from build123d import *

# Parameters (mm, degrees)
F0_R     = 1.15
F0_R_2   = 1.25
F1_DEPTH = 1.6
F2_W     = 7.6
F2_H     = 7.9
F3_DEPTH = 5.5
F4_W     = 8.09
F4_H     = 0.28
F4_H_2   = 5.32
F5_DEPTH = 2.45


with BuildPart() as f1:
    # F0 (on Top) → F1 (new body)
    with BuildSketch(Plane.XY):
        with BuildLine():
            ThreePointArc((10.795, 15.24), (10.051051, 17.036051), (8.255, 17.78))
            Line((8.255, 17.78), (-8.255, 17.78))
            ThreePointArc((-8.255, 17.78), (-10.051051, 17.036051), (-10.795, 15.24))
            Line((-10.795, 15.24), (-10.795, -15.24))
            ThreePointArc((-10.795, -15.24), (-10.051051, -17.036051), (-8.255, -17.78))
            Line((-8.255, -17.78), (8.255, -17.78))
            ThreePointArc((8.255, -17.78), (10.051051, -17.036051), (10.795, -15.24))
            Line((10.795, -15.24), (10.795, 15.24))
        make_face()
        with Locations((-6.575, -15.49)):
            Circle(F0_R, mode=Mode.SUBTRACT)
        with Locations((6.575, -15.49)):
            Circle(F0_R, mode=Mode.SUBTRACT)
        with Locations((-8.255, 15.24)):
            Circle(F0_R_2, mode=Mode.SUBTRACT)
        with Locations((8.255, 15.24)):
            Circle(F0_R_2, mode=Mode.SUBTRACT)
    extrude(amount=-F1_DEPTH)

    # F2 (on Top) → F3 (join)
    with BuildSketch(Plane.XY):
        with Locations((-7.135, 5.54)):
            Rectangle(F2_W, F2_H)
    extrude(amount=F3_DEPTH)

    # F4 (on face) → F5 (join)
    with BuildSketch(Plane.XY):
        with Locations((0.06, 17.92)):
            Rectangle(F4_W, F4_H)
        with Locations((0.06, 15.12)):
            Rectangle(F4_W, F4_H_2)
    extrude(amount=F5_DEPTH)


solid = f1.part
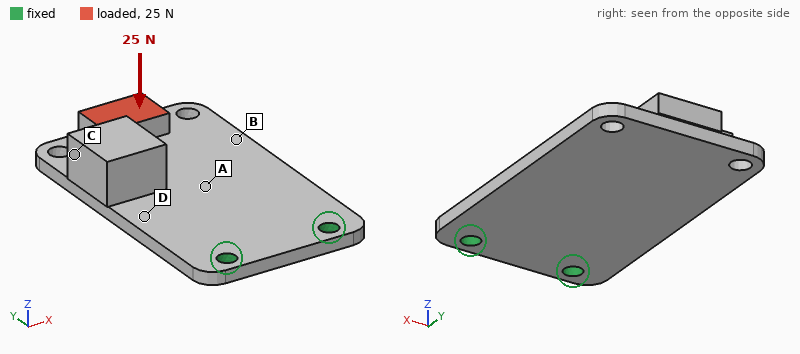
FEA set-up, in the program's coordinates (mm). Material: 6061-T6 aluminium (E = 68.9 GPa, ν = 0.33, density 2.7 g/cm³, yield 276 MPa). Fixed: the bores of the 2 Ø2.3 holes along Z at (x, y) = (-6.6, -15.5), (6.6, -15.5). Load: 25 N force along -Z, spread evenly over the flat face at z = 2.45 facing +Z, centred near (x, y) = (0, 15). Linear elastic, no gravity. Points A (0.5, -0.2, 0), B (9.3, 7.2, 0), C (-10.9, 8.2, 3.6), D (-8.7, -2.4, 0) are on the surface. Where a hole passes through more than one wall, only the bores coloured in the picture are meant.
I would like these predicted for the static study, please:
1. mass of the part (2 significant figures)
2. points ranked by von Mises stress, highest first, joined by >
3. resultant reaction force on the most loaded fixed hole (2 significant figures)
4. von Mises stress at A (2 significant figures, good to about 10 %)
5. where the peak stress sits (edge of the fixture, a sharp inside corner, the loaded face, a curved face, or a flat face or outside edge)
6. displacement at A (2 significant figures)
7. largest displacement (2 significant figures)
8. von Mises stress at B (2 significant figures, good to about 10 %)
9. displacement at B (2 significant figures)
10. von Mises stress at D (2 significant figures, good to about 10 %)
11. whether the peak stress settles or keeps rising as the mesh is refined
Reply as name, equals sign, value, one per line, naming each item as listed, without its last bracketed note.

mass of the part = 4.4 g
points ranked by von Mises stress, highest first, joined by > = D > A > B > C
resultant reaction force on the most loaded fixed hole = 13 N
von Mises stress at A = 38 MPa
where the peak stress sits = edge of the fixture
displacement at A = 0.15 mm
largest displacement = 0.51 mm
von Mises stress at B = 17 MPa
displacement at B = 0.28 mm
von Mises stress at D = 50 MPa
whether the peak stress settles or keeps rising as the mesh is refined = keeps rising
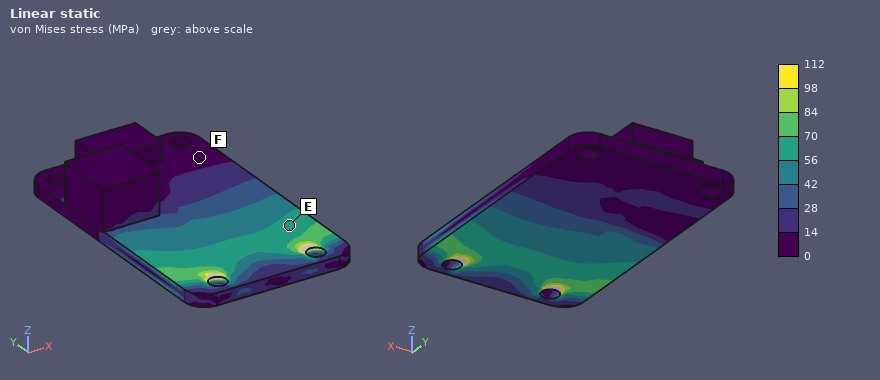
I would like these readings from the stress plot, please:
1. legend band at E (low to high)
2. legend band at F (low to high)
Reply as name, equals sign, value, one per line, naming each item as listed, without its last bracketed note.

legend band at E = 56 to 70 MPa
legend band at F = 0 to 14 MPa
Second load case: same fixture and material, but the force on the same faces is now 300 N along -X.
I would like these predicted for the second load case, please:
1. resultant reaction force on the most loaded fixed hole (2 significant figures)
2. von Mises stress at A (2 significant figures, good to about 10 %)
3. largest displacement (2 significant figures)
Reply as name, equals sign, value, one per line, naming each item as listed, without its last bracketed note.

resultant reaction force on the most loaded fixed hole = 650 N
von Mises stress at A = 92 MPa
largest displacement = 0.26 mm
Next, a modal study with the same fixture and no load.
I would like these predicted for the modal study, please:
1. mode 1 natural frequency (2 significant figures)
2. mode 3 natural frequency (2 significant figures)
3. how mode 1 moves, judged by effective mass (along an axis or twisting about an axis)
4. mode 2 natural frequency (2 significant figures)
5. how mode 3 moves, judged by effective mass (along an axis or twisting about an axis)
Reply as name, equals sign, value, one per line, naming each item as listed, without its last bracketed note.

mode 1 natural frequency = 960 Hz
mode 3 natural frequency = 6800 Hz
how mode 1 moves, judged by effective mass = along Z
mode 2 natural frequency = 3500 Hz
how mode 3 moves, judged by effective mass = along Z
